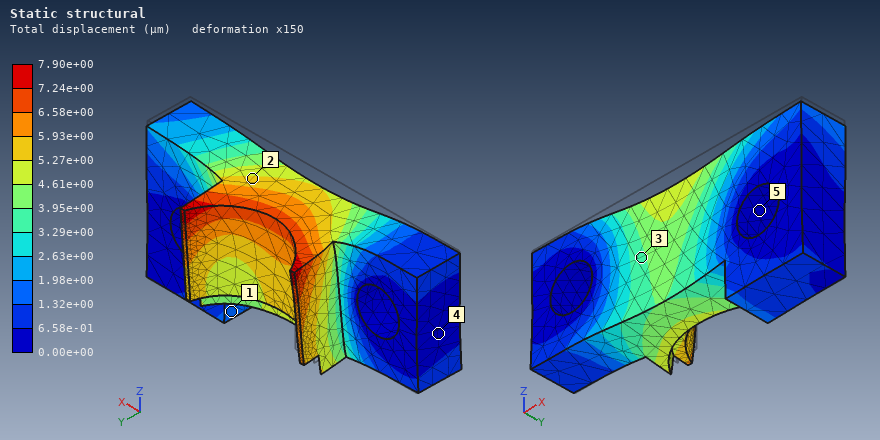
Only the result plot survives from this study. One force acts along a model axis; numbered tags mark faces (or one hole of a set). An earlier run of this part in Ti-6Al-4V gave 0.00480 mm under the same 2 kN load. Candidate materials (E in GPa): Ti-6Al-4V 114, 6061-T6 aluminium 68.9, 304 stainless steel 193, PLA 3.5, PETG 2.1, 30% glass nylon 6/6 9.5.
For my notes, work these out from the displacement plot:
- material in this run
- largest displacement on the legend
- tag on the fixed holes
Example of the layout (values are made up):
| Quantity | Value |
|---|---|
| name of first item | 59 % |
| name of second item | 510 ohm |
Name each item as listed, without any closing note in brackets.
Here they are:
| Quantity | Value |
|---|---|
| material in this run | 6061-T6 aluminium |
| largest displacement on the legend | 7.90e+00 µm |
| tag on the fixed holes | 5 |
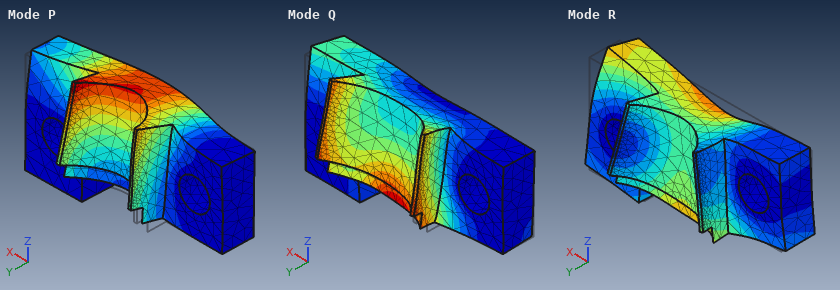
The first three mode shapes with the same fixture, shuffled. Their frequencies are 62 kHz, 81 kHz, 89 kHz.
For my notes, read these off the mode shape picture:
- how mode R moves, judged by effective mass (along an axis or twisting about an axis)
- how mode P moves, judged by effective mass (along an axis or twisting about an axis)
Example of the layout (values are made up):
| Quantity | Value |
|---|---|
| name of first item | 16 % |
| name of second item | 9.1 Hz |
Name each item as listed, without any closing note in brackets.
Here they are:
| Quantity | Value |
|---|---|
| how mode R moves, judged by effective mass | along Z |
| how mode P moves, judged by effective mass | along Y |
